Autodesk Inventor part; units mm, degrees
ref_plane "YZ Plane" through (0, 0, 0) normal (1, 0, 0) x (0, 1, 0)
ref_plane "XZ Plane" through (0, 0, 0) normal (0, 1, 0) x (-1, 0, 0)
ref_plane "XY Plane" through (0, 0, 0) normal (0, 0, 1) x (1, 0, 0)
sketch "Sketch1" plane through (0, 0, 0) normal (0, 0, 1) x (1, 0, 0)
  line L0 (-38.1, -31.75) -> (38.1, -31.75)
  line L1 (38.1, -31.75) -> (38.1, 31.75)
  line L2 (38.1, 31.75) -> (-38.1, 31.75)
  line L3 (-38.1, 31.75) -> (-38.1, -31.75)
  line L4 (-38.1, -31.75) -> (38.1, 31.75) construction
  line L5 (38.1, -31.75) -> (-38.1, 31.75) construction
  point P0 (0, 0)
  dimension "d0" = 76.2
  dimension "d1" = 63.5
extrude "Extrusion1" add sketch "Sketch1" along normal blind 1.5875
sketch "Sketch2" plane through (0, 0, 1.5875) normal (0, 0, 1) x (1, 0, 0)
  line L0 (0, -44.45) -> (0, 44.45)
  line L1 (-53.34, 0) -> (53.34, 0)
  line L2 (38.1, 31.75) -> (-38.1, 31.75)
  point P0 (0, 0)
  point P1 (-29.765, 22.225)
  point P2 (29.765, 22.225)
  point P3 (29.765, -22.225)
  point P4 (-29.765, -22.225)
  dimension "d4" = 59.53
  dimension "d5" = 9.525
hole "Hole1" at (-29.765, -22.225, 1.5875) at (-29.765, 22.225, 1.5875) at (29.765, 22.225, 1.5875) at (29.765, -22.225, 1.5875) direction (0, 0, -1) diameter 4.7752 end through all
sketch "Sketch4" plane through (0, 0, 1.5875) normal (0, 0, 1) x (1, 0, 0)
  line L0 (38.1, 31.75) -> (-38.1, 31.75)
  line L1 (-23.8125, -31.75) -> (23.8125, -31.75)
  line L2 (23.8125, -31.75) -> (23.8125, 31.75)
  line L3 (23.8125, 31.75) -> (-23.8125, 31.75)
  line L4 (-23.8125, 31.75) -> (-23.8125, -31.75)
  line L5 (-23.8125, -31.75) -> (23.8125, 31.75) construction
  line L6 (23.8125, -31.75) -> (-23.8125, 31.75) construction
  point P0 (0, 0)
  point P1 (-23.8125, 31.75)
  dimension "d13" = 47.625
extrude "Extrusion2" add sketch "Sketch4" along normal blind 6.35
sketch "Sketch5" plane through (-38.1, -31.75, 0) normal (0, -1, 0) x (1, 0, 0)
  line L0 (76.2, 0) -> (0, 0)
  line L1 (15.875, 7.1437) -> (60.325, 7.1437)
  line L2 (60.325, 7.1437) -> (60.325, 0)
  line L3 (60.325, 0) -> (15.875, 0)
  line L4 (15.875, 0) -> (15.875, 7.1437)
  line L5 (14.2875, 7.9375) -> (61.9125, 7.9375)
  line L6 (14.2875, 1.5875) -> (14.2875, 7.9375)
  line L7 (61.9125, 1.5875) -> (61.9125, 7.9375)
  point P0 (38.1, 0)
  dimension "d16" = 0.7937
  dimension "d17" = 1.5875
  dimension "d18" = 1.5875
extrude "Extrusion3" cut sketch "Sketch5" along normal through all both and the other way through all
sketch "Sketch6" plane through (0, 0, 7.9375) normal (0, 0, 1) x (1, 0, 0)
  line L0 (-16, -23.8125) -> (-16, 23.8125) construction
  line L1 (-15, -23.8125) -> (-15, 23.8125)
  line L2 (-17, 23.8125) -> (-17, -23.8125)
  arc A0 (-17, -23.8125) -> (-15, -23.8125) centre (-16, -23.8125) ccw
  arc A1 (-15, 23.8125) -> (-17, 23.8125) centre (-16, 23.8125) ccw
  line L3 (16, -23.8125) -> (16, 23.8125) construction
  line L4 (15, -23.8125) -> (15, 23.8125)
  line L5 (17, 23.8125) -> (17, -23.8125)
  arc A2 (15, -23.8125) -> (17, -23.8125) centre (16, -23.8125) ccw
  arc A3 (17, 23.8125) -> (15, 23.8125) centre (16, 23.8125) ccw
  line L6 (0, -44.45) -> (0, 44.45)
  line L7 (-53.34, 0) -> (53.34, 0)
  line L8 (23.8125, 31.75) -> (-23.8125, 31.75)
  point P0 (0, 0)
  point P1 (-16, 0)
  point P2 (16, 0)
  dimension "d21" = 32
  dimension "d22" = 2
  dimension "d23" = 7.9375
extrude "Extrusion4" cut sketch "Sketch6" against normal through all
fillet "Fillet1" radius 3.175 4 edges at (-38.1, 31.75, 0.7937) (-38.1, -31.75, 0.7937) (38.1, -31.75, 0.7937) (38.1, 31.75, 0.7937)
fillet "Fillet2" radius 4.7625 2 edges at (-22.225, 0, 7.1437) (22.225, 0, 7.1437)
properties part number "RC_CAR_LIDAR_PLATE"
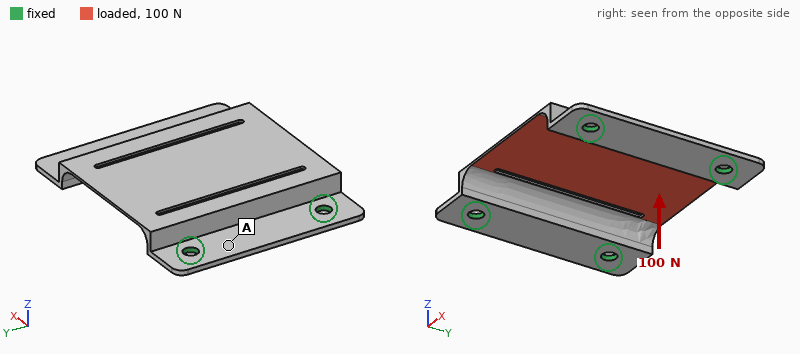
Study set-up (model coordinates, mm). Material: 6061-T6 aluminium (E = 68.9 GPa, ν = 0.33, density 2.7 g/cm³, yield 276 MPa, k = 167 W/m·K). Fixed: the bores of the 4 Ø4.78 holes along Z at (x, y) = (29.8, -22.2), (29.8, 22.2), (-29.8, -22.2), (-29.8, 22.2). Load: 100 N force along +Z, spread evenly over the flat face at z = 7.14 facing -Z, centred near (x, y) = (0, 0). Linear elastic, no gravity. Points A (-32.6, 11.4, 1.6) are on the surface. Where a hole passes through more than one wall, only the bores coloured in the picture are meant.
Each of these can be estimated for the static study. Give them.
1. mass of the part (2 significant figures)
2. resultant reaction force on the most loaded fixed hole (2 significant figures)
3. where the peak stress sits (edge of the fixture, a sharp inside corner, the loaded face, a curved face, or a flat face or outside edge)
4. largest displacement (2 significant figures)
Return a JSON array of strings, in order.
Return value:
["19 g", "50 N", "a curved face", "0.81 mm"]
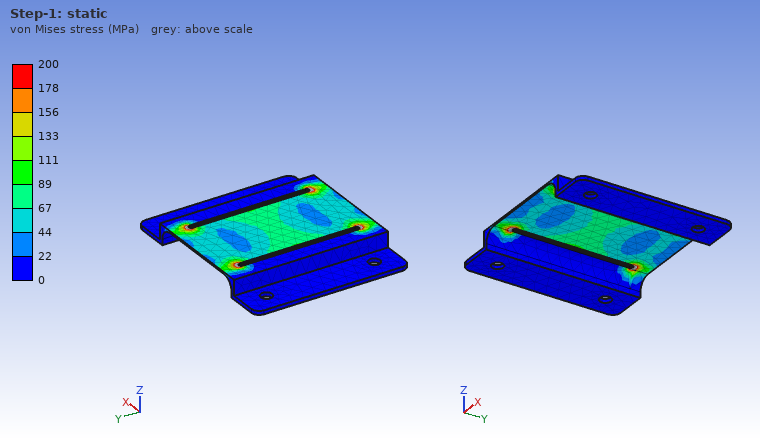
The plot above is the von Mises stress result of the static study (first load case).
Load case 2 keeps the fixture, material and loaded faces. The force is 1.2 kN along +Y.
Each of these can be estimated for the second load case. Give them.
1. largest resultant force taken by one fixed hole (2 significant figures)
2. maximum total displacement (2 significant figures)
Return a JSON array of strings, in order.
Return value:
["330 N", "80 µm"]
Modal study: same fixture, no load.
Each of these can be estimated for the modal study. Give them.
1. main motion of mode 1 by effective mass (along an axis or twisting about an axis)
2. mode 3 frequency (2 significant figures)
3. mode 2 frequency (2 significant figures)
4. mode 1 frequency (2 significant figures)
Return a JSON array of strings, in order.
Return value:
["along Z", "2300 Hz", "2000 Hz", "970 Hz"]
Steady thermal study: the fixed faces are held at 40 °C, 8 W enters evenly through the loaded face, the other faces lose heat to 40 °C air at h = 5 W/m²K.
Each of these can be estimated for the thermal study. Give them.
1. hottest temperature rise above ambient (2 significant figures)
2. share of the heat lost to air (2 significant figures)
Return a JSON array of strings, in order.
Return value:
["31 K", "4.3 %"]
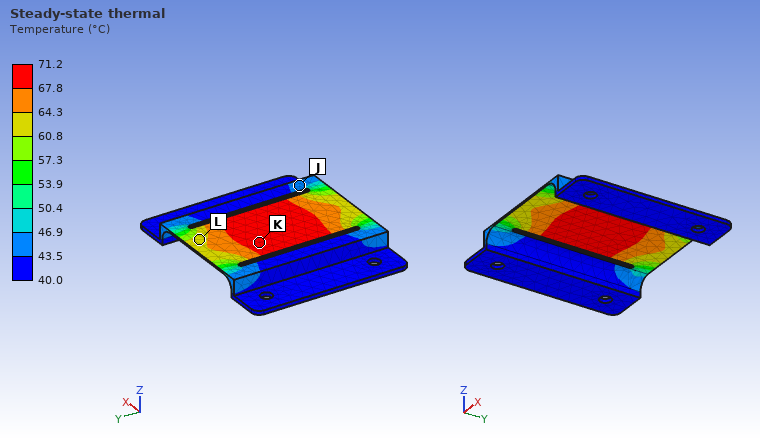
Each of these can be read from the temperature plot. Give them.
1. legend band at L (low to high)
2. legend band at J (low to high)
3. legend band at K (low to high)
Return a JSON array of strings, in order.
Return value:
["60.8 to 64.3 °C", "43.5 to 46.9 °C", "67.8 to 71.2 °C"]
